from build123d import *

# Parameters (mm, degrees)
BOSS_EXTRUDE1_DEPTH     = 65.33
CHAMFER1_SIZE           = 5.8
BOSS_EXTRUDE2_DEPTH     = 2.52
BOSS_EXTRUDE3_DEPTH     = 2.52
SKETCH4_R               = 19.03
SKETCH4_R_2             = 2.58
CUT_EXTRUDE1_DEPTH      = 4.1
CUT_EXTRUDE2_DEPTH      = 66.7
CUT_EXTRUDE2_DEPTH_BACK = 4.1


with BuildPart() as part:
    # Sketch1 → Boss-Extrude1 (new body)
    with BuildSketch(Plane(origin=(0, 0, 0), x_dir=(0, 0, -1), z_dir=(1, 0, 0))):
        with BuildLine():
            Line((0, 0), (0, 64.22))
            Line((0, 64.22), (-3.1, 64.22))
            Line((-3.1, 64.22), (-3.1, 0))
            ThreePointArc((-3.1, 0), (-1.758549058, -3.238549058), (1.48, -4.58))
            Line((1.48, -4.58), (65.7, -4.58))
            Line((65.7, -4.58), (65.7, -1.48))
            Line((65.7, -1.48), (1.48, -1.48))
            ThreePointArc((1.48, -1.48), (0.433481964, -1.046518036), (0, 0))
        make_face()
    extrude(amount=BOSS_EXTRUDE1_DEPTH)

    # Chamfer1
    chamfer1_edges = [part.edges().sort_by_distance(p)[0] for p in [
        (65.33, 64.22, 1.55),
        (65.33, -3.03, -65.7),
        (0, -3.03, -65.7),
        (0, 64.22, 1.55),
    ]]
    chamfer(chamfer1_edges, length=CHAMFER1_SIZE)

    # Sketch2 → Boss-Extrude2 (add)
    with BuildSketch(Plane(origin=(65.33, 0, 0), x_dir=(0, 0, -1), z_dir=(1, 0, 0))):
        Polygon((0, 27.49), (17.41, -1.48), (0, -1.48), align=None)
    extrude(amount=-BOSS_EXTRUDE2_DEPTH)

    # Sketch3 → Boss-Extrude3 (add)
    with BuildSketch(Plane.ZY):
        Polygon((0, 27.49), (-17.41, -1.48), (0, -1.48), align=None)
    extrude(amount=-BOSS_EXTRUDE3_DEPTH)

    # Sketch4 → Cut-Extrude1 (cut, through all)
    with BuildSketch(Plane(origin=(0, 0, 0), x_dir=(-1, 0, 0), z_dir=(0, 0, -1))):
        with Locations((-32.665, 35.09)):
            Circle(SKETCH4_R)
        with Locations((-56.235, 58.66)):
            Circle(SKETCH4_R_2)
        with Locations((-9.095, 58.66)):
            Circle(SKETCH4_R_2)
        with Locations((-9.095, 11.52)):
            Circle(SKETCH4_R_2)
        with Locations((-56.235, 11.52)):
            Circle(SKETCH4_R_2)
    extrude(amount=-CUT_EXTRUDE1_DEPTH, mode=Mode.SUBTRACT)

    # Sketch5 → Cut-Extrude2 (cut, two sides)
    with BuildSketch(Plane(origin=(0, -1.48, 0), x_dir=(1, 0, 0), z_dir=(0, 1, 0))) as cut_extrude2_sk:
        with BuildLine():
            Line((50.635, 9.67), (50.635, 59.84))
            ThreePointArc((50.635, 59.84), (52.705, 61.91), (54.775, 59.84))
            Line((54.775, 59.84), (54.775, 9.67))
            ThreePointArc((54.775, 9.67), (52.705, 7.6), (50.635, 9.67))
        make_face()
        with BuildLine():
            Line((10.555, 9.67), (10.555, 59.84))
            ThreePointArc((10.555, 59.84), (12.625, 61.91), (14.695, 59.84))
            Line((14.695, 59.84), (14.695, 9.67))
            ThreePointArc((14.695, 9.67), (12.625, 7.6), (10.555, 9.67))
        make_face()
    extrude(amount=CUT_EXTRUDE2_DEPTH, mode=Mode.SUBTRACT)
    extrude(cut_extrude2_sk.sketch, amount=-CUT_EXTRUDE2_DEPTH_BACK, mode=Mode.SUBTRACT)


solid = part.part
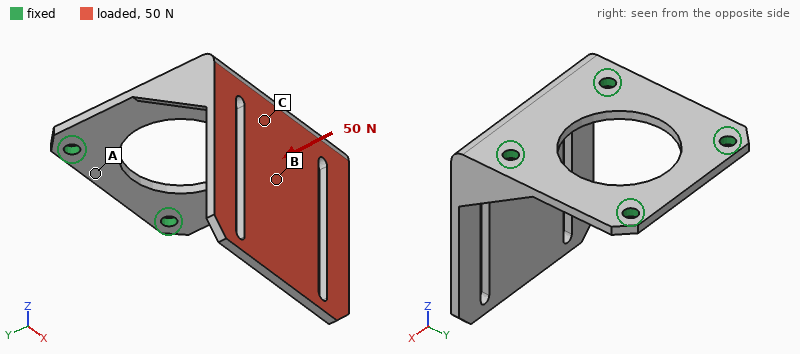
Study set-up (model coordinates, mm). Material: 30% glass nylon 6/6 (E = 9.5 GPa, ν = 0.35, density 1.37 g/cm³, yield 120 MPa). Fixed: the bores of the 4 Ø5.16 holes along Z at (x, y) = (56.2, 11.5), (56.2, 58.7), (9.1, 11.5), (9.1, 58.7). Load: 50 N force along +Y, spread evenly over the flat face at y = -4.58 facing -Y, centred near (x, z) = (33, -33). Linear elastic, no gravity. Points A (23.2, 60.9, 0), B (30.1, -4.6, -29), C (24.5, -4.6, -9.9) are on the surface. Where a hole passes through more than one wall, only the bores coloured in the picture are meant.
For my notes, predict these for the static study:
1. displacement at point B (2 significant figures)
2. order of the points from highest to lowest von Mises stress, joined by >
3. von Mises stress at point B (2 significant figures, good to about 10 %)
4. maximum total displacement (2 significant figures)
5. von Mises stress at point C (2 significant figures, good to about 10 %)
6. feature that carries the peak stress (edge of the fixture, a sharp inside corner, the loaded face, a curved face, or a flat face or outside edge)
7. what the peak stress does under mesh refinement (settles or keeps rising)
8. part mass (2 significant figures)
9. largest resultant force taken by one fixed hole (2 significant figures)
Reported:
0.45 mm
C > B > A
3.3 MPa
1.3 mm
7.4 MPa
edge of the fixture
keeps rising
31 g
28 N
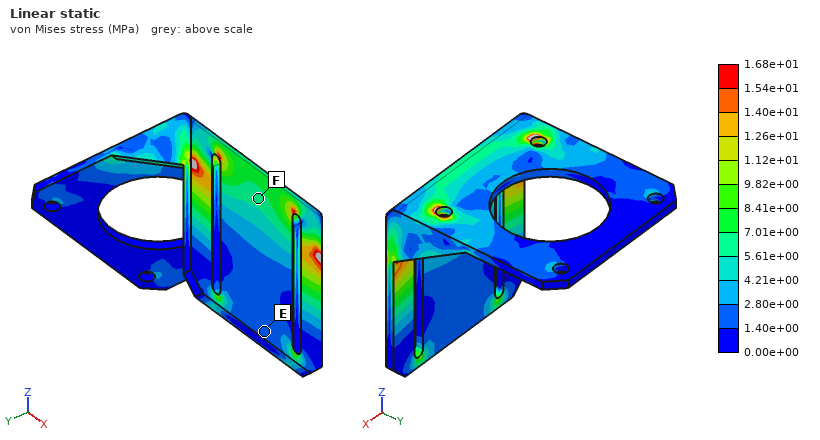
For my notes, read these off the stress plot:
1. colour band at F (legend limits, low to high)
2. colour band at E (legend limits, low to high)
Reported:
5.61e+00 to 7.01e+00 MPa
1.40e+00 to 2.80e+00 MPa
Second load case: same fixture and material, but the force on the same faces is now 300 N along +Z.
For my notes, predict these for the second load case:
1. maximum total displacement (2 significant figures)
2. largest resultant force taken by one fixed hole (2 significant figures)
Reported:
1.1 mm
170 N
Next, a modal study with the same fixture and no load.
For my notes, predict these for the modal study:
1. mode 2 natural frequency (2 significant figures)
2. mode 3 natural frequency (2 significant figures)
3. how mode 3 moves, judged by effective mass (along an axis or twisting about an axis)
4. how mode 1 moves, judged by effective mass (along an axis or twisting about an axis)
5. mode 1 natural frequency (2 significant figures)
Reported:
800 Hz
1200 Hz
along X
along Y
320 Hz
